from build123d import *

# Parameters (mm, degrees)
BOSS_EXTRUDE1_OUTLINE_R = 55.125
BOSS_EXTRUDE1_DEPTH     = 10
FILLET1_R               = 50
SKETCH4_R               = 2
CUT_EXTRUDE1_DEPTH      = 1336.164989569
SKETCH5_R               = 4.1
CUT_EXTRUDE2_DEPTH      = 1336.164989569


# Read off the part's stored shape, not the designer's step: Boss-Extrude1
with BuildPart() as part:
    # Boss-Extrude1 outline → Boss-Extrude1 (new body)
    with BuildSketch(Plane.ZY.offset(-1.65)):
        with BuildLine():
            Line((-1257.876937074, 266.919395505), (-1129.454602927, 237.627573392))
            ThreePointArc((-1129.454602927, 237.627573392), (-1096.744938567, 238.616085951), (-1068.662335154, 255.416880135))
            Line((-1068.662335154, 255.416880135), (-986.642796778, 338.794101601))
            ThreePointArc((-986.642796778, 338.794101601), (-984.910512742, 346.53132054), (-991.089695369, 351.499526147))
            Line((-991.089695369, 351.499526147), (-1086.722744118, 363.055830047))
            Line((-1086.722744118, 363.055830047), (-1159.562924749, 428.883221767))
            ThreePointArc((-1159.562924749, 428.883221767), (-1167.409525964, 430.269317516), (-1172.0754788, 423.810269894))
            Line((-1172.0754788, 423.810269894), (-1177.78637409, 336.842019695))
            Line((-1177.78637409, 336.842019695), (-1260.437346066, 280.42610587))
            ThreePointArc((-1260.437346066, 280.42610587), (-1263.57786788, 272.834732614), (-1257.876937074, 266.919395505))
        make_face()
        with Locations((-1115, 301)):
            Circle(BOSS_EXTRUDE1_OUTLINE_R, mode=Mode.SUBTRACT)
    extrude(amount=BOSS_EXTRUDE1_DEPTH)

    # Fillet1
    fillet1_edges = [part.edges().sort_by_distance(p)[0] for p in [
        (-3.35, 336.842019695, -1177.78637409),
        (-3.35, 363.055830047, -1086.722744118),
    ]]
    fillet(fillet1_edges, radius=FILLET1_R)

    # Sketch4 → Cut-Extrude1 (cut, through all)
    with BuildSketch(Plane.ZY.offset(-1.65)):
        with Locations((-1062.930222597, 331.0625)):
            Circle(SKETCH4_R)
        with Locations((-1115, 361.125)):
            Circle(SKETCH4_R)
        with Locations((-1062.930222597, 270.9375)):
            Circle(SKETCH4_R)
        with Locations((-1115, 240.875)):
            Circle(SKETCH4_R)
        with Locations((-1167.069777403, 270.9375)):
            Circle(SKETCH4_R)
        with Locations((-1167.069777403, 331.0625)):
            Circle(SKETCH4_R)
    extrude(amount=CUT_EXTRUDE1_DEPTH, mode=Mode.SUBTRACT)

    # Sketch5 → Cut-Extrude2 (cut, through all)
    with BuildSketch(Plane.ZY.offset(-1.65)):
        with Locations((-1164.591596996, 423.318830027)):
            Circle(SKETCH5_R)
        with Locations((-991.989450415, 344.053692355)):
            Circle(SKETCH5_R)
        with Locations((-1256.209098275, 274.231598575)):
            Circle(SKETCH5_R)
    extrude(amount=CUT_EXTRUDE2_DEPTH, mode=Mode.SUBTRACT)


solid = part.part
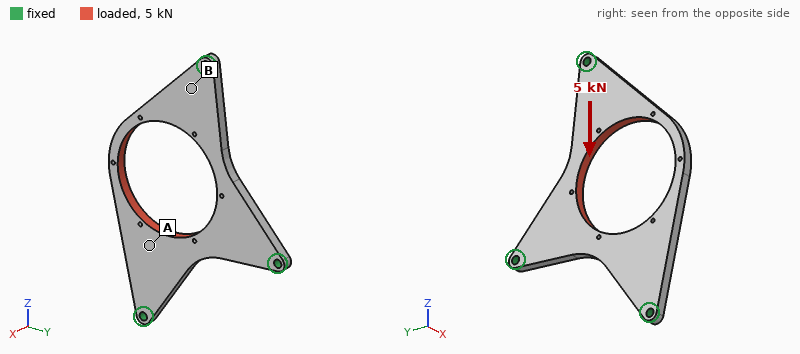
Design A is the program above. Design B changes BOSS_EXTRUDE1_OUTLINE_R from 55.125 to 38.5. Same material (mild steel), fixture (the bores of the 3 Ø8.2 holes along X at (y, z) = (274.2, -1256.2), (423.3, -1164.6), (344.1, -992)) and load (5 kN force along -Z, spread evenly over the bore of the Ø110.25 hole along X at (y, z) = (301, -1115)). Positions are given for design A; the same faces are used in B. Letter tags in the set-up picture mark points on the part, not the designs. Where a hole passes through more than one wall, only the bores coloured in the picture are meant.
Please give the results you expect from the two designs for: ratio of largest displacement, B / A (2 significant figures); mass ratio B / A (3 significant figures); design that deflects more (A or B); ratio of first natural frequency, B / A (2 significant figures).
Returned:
0.32
1.31
A
0.84
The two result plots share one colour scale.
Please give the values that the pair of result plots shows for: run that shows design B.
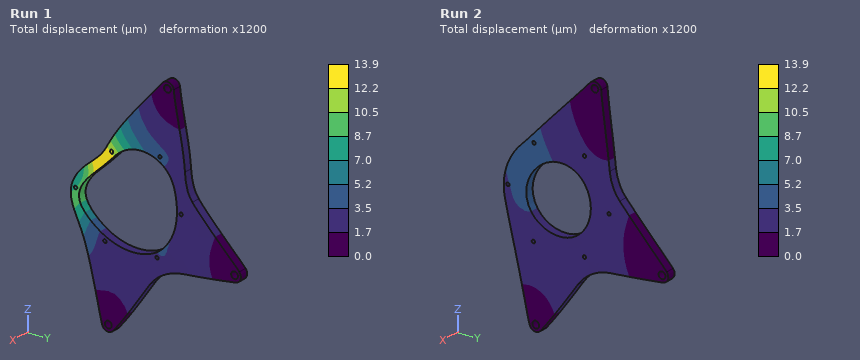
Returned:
Run 2
